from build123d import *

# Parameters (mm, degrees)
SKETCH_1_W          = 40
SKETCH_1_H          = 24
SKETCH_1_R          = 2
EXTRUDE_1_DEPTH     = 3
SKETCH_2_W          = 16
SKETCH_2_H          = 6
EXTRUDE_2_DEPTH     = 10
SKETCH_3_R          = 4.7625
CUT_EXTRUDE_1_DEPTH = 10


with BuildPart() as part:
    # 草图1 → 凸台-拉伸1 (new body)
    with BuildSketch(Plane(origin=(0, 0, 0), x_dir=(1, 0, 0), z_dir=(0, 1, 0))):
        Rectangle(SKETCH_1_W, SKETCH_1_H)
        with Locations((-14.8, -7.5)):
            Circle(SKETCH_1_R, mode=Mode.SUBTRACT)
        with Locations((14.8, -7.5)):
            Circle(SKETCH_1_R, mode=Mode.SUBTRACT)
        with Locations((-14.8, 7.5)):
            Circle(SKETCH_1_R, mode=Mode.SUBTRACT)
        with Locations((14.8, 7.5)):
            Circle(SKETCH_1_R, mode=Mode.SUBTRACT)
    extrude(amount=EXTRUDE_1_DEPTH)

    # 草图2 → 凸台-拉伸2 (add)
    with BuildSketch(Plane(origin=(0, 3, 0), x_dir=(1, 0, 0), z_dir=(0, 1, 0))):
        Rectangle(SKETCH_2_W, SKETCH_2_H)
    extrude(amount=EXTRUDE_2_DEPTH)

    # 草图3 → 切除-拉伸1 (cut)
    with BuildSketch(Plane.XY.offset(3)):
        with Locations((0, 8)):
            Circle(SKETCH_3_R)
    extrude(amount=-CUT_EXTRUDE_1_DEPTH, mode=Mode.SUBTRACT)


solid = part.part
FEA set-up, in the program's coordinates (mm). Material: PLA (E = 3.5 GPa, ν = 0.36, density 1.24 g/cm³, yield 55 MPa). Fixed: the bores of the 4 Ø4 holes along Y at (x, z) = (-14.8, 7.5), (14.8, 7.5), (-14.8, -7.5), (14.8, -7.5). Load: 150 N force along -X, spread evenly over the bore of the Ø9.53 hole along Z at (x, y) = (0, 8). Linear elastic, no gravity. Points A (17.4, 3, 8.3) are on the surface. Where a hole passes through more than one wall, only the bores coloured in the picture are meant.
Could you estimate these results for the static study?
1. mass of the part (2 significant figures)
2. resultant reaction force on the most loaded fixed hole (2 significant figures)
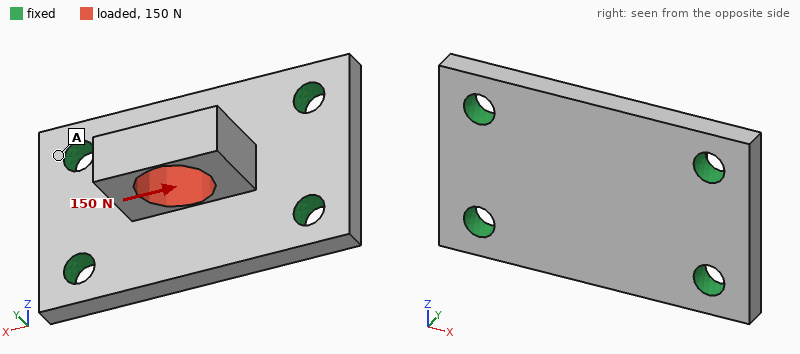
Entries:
4.0 g
45 N
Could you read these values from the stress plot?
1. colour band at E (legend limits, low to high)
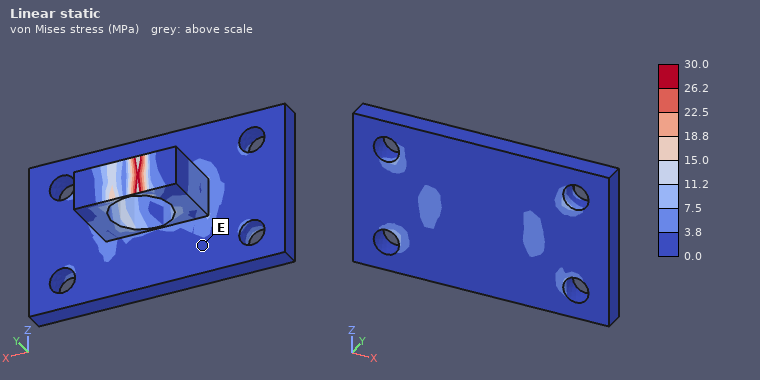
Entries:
0.0 to 3.8 MPa
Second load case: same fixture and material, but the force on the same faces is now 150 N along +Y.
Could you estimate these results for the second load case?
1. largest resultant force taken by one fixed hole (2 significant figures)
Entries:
39 N
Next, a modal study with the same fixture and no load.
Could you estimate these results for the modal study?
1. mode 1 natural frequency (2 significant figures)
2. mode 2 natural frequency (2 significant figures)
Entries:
6100 Hz
6200 Hz
